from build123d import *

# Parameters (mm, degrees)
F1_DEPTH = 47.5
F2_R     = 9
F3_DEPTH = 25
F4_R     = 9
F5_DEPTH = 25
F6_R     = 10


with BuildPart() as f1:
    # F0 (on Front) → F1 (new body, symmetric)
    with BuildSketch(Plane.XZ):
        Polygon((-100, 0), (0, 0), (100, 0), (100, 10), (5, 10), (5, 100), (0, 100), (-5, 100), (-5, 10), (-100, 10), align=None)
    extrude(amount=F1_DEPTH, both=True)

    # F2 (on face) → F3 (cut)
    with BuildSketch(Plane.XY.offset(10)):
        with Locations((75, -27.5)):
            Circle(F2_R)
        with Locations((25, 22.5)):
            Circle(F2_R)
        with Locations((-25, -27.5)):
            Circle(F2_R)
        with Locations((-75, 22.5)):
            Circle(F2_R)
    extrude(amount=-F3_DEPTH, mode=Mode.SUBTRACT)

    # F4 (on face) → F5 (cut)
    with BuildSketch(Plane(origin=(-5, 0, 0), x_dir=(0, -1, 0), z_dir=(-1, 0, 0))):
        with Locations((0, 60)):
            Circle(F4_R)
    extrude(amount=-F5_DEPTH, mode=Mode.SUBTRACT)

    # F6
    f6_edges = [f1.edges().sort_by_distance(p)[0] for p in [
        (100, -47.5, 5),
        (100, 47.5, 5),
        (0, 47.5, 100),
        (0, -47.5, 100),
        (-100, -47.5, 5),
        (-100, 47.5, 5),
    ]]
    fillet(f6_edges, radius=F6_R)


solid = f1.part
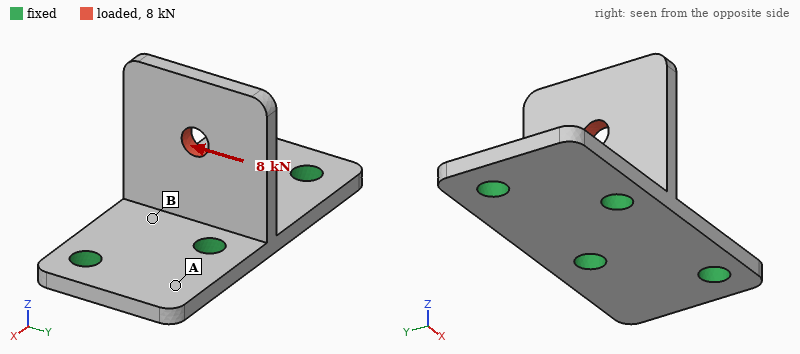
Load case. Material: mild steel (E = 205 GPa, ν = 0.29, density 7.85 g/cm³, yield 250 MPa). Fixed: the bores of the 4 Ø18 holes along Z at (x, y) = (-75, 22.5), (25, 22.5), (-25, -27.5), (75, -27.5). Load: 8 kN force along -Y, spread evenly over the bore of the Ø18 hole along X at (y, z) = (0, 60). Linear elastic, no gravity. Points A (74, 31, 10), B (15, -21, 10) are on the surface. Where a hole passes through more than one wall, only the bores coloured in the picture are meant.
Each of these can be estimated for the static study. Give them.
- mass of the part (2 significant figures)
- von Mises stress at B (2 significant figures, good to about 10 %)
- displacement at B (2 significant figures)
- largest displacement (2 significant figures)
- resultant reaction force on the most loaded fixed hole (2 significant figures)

2.1 kg
28 MPa
13 µm
79 µm
6.5 kN
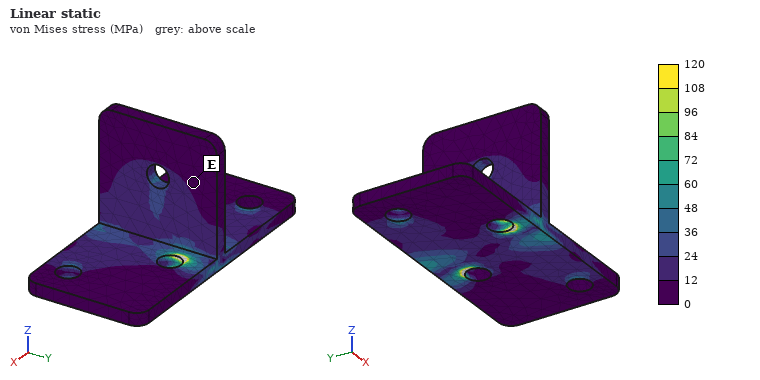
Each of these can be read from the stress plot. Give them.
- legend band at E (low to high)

0 to 12 MPa
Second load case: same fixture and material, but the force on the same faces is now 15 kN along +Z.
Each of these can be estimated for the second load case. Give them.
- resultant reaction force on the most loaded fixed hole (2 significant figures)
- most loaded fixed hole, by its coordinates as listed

7.5 kN
(25, 22.5)
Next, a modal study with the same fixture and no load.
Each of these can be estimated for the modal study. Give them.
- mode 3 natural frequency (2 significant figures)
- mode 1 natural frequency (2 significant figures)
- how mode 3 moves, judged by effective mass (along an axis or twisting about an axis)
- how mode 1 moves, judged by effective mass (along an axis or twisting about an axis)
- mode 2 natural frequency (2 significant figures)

2600 Hz
890 Hz
along Y
along X
2100 Hz
